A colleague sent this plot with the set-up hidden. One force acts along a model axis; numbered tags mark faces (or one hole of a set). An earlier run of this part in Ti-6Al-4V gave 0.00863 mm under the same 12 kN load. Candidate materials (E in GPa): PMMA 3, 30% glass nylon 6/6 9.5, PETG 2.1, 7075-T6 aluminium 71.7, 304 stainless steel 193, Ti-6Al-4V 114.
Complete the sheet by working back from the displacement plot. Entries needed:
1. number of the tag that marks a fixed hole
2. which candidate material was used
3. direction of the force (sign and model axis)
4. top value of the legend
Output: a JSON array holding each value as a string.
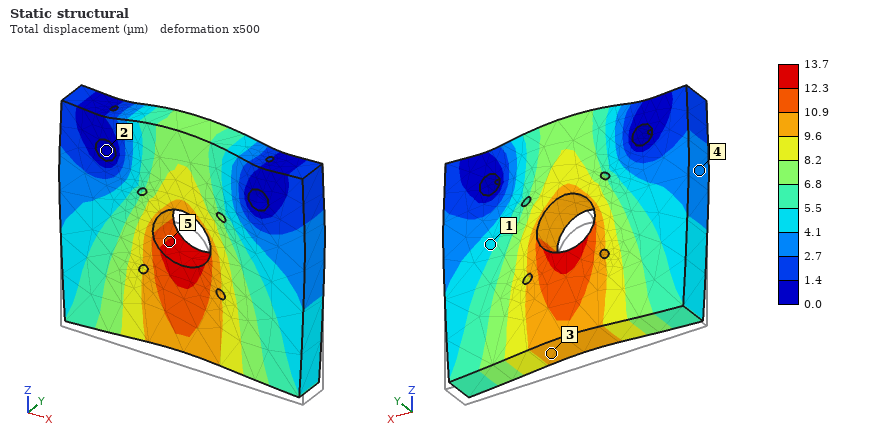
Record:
["2", "7075-T6 aluminium", "+Z", "13.7 µm"]
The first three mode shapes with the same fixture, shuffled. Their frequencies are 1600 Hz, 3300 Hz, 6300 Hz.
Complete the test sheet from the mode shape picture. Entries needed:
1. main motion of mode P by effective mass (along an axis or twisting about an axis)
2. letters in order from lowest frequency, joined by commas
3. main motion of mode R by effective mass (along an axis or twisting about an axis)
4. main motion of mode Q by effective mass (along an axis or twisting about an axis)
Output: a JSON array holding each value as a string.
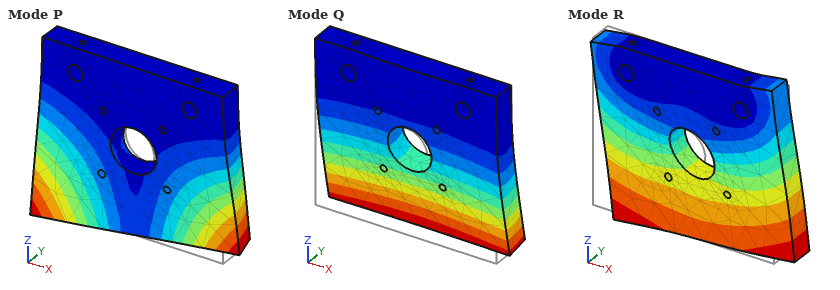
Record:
["twisting about Z", "Q, P, R", "along X", "along Y"]
